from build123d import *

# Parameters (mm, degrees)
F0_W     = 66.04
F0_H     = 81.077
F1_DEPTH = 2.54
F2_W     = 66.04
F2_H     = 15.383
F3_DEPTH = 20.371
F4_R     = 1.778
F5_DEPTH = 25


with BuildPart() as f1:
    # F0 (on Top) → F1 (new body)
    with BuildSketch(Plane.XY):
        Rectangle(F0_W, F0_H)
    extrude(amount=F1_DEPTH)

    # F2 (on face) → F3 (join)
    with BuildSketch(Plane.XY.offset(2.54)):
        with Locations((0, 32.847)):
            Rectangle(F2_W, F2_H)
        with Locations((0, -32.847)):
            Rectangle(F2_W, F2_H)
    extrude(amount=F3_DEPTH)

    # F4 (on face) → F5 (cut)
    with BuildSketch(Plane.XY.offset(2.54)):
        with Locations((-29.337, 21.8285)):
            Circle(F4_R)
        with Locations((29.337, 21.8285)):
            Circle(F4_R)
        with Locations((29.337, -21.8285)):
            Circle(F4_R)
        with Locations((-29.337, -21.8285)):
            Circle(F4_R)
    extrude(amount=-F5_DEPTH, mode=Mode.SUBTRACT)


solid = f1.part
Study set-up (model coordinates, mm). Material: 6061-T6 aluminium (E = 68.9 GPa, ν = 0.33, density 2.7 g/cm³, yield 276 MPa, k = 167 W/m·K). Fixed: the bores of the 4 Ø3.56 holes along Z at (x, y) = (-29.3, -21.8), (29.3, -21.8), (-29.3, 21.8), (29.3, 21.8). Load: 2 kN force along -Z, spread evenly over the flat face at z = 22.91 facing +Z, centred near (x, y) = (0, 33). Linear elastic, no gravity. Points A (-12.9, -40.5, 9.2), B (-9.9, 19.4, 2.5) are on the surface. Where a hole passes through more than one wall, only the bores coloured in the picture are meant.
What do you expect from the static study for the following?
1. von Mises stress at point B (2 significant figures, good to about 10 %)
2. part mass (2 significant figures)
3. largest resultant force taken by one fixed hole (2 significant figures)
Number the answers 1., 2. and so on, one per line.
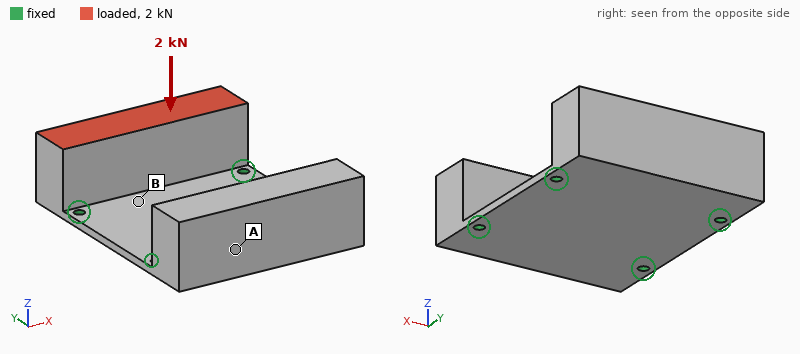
1. 94 MPa
2. 150 g
3. 1.1 kN
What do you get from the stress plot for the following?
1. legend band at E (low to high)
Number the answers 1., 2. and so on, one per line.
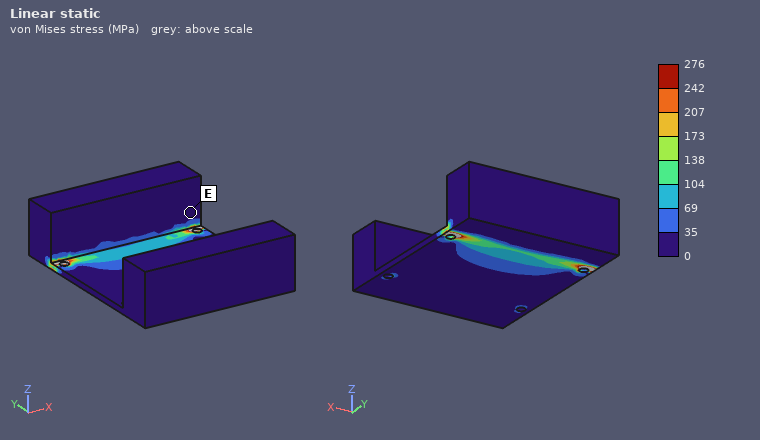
1. 0 to 35 MPa
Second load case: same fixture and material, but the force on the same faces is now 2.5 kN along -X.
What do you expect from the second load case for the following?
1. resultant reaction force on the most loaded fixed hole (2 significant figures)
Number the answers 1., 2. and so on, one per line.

1. 1.6 kN
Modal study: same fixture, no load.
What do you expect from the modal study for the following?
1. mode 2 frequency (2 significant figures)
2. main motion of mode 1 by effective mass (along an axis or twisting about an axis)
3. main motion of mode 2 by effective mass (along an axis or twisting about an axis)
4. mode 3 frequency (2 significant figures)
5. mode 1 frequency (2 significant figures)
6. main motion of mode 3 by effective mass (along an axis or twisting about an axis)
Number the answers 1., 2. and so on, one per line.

1. 1300 Hz
2. along Z
3. along Y
4. 5400 Hz
5. 1200 Hz
6. along Z
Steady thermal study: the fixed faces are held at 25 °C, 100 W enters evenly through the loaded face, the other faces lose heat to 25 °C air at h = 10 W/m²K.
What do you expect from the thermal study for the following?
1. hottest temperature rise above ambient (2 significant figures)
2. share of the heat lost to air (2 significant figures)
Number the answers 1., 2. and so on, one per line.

1. 58 K
2. 3.5 %
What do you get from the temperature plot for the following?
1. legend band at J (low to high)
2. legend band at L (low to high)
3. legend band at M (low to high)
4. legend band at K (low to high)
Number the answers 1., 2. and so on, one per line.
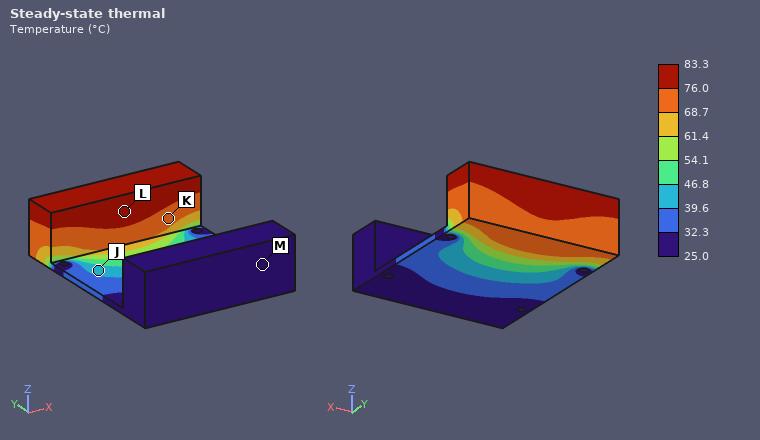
1. 39.6 to 46.8 °C
2. 76.0 to 83.3 °C
3. 25.0 to 32.3 °C
4. 68.7 to 76.0 °C
